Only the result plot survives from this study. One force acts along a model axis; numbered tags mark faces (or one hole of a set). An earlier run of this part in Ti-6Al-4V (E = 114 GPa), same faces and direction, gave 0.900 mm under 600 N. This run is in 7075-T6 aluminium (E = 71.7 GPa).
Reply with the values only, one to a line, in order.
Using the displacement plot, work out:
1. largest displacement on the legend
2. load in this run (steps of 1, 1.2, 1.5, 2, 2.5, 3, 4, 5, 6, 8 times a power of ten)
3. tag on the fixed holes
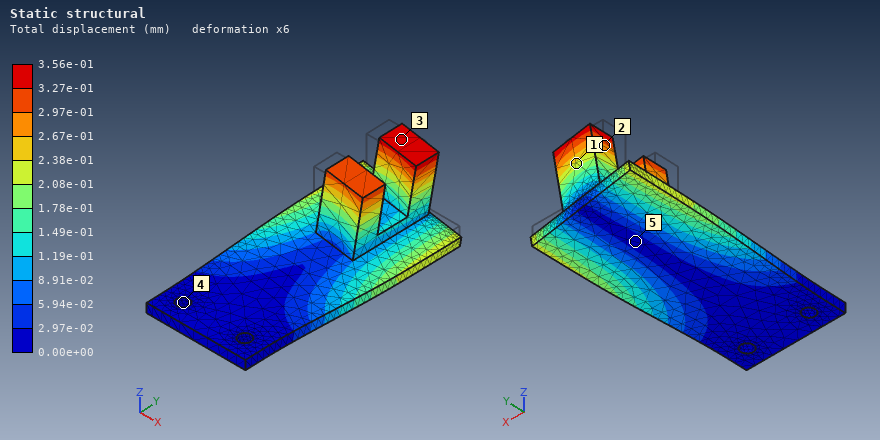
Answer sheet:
3.56e-01 mm
150 N
4
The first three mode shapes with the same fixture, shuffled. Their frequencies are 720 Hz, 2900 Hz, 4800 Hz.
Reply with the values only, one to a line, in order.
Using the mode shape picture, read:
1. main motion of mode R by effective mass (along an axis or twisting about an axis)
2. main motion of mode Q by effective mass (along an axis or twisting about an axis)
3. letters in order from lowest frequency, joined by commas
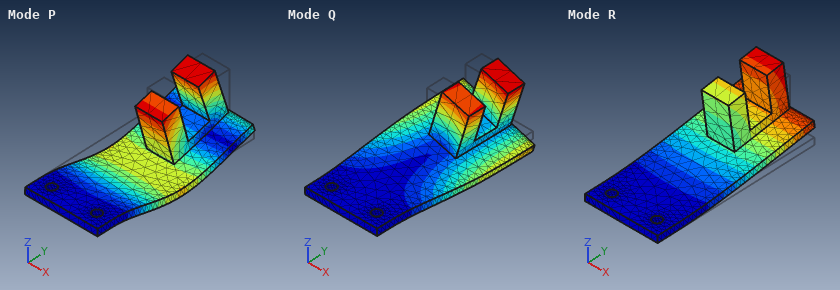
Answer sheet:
along Z
along X
R, Q, P
